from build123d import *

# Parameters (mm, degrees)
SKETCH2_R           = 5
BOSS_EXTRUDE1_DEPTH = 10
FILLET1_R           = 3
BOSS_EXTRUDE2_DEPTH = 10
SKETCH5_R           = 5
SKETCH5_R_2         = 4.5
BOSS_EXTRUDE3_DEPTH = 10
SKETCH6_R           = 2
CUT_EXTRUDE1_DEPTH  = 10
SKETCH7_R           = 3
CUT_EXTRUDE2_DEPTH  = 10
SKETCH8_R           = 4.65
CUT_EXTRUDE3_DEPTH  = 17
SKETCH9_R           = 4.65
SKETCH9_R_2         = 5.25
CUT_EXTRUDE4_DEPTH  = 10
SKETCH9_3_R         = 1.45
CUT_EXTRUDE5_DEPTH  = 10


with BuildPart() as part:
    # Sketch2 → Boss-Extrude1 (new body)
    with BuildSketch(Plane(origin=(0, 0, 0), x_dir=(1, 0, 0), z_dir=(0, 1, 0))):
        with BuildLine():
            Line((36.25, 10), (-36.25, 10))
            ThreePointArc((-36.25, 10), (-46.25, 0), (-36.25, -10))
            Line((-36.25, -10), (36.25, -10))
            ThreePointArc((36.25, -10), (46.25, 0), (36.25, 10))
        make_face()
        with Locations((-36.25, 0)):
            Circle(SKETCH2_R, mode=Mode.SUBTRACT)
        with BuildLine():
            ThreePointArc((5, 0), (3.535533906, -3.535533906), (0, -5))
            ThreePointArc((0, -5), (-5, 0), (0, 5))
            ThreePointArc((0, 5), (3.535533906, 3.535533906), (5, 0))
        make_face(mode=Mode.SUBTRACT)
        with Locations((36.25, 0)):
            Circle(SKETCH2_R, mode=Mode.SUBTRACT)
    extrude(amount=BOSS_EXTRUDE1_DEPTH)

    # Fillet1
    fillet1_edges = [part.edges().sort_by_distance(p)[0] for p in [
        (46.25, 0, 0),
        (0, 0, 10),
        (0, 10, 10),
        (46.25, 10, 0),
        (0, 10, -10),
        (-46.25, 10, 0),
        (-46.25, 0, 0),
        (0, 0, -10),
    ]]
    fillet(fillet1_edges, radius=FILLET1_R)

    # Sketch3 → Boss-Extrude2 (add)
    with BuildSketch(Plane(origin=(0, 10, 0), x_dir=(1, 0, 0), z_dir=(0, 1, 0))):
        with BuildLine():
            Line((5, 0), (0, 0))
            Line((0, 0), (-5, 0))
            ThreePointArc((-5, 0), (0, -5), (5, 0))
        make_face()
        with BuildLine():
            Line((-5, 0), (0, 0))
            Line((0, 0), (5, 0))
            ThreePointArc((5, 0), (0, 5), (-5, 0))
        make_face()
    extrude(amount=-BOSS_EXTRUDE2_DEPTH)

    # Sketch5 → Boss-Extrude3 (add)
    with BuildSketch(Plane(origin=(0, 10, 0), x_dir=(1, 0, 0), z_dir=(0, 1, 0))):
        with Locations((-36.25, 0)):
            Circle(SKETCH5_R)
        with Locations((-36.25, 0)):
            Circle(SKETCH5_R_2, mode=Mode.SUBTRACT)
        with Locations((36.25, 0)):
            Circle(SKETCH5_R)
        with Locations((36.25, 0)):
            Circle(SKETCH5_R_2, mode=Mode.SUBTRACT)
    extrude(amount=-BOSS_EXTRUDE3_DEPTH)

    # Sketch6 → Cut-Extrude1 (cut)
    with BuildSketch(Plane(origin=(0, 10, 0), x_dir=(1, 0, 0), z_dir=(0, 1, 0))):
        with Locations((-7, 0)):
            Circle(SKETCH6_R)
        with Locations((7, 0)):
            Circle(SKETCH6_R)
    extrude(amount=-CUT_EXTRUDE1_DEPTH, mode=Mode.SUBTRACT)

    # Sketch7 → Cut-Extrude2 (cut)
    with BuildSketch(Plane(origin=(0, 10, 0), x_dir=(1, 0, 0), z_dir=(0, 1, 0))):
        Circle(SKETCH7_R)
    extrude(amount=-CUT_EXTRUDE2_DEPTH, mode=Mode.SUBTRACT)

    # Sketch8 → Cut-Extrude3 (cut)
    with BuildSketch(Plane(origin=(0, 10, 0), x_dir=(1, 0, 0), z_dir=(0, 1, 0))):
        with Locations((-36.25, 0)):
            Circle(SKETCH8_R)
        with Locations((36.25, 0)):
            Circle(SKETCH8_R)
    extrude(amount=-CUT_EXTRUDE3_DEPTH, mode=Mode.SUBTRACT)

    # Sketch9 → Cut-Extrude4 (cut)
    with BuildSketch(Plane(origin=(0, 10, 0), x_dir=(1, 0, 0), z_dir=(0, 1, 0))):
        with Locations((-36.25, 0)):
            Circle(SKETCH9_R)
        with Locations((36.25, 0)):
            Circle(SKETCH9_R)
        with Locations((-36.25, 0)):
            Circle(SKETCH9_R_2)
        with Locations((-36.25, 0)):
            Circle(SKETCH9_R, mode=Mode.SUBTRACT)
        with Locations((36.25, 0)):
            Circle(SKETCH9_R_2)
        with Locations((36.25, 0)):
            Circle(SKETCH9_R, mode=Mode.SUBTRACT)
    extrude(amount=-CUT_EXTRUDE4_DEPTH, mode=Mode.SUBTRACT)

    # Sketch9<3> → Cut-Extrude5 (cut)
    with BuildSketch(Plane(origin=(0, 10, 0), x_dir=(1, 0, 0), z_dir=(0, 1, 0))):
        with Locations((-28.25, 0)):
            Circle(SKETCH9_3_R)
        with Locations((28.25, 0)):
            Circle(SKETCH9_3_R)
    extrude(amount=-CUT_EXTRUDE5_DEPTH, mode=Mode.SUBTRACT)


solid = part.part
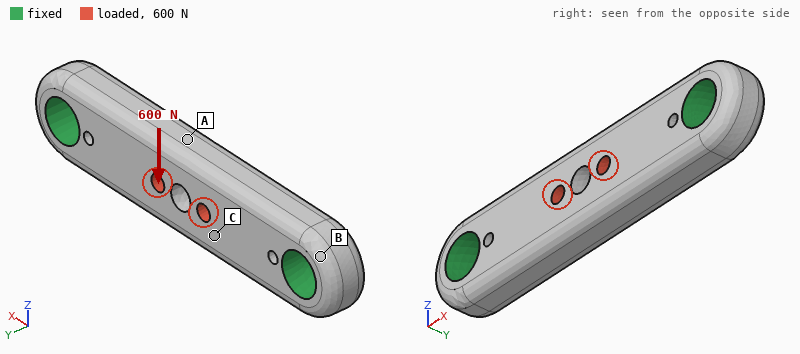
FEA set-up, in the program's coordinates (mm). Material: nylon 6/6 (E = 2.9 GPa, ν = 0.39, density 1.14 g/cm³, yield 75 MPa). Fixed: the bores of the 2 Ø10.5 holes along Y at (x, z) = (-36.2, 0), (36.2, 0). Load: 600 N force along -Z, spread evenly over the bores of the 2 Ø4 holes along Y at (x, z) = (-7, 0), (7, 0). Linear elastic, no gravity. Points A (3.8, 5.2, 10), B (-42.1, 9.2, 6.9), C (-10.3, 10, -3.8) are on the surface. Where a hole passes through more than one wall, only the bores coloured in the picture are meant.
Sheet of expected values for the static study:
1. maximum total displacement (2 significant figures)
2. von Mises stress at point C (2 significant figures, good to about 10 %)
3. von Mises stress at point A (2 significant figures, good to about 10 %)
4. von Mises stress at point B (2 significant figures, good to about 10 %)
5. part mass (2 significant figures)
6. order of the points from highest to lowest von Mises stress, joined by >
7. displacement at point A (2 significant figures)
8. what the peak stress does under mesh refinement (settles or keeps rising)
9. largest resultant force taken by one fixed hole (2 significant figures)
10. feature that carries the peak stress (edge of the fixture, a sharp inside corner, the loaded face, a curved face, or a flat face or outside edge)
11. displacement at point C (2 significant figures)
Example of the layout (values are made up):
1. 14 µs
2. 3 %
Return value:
1. 0.12 mm
2. 3.5 MPa
3. 7.2 MPa
4. 1.1 MPa
5. 16 g
6. A > C > B
7. 0.11 mm
8. keeps rising
9. 300 N
10. edge of the fixture
11. 0.095 mm
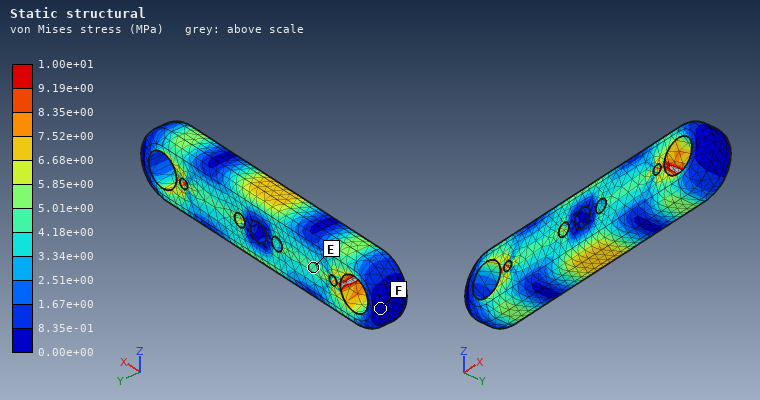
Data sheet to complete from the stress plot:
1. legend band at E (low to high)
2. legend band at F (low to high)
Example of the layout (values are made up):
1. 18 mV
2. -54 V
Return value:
1. 4.18e+00 to 5.01e+00 MPa
2. 0.00e+00 to 8.35e-01 MPa
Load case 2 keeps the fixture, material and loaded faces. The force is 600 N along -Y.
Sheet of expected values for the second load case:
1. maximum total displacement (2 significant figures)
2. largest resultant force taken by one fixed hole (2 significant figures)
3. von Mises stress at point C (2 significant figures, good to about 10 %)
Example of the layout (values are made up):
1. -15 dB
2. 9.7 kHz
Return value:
1. 0.25 mm
2. 300 N
3. 6.9 MPa
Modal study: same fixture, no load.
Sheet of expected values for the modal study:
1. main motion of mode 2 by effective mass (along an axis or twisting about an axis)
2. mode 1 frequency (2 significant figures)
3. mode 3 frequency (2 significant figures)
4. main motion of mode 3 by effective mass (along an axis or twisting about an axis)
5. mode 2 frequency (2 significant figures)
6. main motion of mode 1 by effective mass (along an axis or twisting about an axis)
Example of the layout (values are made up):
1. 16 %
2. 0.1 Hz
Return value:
1. along Z
2. 3200 Hz
3. 5800 Hz
4. twisting about X
5. 4500 Hz
6. along Y
